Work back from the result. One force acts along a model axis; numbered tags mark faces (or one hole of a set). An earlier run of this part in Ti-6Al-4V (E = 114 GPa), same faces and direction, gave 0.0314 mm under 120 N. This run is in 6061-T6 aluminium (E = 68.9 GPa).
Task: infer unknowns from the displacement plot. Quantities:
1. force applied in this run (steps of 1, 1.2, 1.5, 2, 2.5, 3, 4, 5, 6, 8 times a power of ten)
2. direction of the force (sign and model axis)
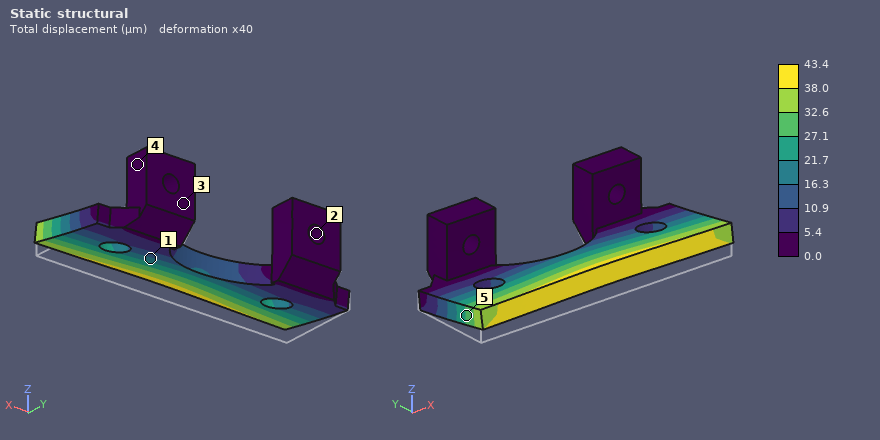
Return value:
100 N
+Z
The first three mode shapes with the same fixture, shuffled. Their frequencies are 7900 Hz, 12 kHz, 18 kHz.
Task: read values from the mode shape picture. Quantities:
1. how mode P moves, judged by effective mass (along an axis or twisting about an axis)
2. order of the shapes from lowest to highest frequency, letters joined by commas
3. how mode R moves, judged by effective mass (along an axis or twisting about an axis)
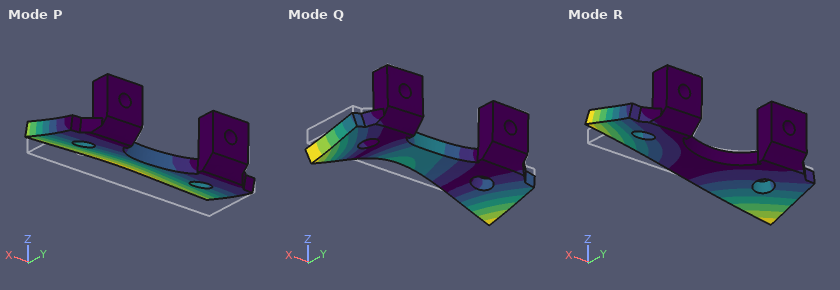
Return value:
along Z
P, R, Q
twisting about Y
